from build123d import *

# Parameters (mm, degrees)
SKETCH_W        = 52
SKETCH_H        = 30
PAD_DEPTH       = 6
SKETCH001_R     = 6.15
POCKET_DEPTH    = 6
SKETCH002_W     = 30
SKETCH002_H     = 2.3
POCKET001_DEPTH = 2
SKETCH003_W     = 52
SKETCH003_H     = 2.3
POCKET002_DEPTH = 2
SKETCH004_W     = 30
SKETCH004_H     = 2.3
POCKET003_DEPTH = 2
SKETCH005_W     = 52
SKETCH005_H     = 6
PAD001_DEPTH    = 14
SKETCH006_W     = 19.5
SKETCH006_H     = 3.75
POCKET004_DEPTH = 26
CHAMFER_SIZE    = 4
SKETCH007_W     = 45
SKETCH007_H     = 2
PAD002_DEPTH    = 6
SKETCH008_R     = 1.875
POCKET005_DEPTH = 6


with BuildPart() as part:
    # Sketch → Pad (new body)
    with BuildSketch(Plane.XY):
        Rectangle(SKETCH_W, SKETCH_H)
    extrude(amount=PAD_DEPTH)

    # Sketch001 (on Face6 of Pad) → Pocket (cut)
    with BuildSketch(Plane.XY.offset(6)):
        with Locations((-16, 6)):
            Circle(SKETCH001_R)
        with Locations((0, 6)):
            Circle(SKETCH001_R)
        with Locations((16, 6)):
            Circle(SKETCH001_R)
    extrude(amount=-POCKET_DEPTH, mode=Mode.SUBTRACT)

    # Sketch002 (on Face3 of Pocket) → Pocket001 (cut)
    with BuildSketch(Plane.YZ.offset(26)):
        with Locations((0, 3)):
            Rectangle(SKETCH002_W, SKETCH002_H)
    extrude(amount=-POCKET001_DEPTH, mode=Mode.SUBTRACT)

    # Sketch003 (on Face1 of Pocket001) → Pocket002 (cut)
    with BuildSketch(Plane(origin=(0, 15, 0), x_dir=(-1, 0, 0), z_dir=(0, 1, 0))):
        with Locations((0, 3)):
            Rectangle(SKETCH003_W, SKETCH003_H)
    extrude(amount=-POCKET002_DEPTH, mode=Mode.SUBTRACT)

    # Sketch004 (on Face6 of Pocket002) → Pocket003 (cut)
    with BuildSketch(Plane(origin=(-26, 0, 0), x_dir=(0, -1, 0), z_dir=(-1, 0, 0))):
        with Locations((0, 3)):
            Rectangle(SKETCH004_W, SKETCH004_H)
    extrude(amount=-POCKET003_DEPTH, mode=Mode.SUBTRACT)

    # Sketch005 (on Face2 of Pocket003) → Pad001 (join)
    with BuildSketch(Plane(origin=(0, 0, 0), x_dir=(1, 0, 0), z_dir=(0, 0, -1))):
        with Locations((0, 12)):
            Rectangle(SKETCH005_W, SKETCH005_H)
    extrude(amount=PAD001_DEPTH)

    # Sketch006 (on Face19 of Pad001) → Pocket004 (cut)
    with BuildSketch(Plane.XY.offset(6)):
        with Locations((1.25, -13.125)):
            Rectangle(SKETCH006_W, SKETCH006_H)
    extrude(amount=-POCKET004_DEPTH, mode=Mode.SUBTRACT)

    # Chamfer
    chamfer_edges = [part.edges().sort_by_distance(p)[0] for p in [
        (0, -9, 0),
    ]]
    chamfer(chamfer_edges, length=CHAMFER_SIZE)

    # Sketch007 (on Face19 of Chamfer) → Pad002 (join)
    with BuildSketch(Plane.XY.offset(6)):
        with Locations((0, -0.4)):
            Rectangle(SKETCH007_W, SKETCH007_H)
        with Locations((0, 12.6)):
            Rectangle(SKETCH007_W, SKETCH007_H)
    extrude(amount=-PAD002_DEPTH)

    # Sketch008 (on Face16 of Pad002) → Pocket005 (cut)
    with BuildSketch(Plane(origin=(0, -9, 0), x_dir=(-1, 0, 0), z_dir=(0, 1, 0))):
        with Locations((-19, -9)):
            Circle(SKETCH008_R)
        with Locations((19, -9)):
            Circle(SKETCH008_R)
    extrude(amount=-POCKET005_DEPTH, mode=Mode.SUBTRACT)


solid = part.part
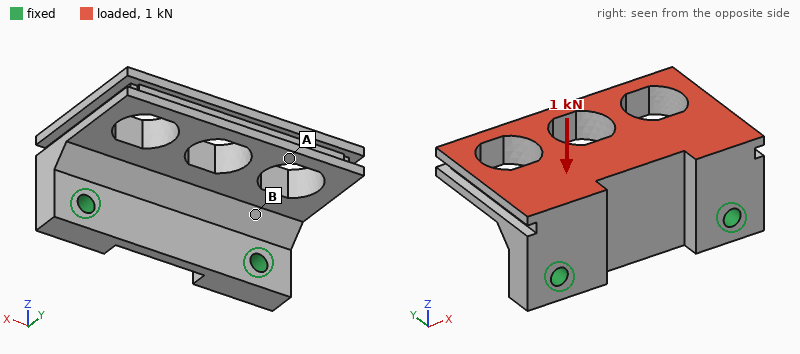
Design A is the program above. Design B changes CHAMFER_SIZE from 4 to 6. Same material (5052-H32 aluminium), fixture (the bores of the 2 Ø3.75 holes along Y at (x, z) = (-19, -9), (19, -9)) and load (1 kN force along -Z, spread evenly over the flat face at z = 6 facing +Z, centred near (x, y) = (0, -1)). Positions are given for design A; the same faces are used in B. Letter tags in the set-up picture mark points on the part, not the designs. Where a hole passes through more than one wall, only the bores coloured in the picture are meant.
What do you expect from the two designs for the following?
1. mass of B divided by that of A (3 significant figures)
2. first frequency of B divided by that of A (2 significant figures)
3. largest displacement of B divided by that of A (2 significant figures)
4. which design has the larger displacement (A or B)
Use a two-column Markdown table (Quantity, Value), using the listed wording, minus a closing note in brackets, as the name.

| Quantity | Value |
|---|---|
| mass of B divided by that of A | 1.05 |
| first frequency of B divided by that of A | 1.1 |
| largest displacement of B divided by that of A | 0.82 |
| which design has the larger displacement | A |
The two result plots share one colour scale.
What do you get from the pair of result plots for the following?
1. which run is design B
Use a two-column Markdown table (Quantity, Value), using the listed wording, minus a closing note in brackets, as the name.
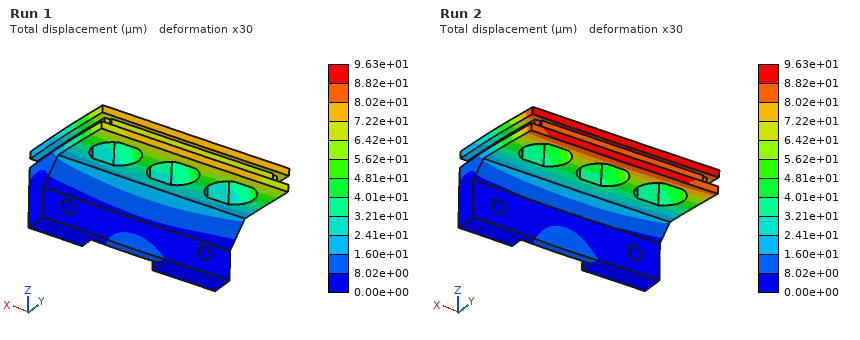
| Quantity | Value |
|---|---|
| which run is design B | Run 1 |
